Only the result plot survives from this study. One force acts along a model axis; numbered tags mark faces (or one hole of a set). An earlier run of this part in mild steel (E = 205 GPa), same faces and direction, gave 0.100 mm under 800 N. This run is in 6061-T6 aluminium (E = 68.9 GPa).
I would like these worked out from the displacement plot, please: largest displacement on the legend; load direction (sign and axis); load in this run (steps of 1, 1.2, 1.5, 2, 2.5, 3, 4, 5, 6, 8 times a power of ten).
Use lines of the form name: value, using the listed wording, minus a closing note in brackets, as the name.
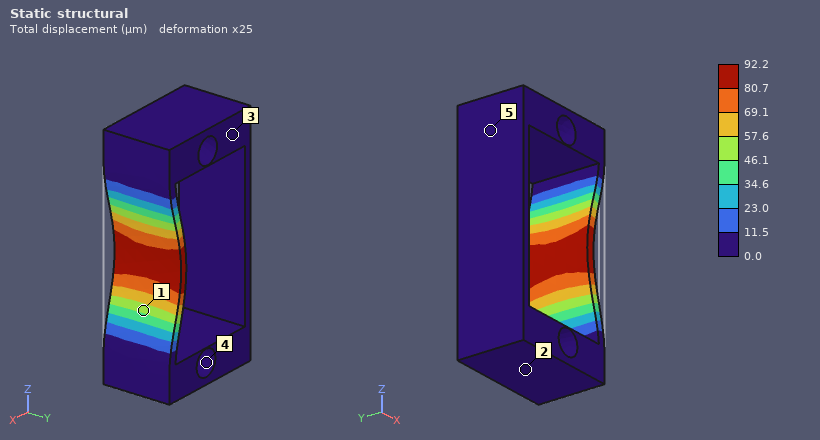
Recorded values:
largest displacement on the legend: 92.2 µm
load direction: -X
load in this run: 250 N
